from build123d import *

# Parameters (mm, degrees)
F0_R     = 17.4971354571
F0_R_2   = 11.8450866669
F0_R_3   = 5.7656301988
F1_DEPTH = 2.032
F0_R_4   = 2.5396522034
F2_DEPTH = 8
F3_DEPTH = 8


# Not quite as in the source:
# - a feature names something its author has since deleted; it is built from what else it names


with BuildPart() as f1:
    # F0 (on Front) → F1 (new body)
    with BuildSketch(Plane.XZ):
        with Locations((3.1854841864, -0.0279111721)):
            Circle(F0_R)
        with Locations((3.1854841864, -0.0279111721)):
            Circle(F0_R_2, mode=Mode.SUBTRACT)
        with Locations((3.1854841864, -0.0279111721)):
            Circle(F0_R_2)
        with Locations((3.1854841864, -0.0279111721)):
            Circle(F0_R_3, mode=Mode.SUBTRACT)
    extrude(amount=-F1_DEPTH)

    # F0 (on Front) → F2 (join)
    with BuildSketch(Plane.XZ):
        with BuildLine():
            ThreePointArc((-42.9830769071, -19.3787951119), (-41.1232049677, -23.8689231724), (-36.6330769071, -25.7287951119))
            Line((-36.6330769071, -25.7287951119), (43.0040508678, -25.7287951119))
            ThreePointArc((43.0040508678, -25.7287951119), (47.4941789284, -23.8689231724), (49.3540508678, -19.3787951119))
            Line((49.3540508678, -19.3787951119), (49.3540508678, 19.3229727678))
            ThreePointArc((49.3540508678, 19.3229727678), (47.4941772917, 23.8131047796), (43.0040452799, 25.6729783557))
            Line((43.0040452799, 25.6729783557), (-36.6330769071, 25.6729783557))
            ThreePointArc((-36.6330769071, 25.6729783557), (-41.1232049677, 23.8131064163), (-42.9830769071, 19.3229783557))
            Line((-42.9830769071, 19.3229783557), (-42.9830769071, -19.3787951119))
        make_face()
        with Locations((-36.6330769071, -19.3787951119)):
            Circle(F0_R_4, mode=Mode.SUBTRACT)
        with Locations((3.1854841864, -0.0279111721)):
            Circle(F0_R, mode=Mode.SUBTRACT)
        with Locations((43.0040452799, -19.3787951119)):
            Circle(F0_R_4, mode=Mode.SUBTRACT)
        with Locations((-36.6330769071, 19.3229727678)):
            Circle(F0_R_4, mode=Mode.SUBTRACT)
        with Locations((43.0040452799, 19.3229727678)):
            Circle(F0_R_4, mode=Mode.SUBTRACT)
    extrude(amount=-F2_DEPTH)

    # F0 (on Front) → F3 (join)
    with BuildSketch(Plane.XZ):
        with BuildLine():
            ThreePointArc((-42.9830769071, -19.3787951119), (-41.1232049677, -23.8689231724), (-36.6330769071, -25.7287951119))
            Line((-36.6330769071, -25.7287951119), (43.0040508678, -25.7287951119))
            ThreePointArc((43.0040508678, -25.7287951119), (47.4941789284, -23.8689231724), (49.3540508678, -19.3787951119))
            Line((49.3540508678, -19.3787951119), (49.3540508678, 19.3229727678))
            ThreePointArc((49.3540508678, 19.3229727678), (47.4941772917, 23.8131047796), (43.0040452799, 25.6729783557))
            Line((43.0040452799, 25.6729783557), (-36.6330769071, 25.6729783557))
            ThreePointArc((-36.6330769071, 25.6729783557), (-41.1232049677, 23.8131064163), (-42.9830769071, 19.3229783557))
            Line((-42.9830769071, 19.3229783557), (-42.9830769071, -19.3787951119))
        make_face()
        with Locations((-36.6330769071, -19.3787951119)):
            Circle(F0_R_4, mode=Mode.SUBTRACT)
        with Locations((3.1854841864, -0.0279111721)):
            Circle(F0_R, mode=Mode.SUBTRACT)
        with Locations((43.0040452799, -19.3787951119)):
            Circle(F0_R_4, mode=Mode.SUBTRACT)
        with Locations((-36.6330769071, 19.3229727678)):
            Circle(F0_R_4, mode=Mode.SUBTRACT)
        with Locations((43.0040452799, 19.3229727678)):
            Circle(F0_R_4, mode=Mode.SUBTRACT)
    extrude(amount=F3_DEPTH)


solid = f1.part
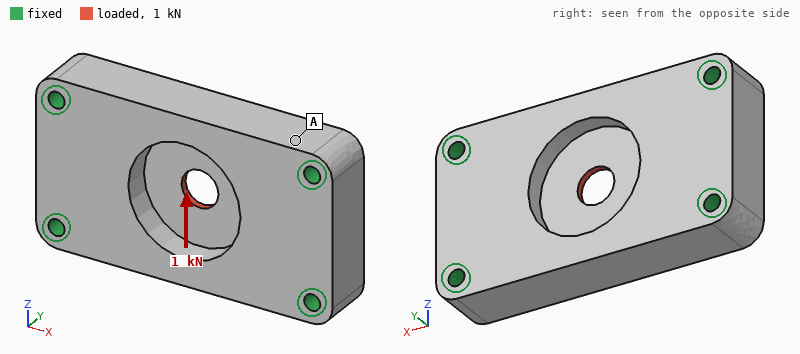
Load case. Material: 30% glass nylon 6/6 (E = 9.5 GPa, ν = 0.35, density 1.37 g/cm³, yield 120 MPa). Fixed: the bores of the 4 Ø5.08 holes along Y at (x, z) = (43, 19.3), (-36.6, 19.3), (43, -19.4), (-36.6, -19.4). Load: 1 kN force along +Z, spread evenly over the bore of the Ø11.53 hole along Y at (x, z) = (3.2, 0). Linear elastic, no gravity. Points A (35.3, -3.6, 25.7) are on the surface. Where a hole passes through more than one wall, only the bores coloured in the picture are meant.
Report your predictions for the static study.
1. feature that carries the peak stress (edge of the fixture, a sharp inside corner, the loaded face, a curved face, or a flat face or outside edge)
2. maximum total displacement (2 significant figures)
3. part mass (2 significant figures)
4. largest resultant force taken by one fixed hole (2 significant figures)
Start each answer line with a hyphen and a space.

- the loaded face
- 25 µm
- 83 g
- 350 N
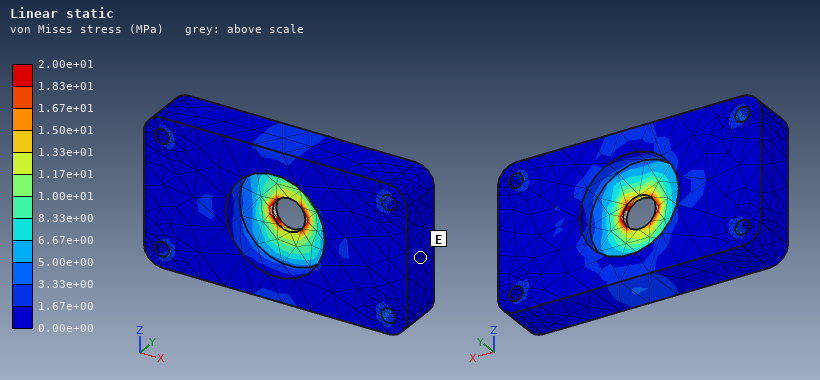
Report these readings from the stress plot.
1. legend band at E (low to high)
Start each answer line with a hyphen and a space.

- 0.00e+00 to 1.67e+00 MPa
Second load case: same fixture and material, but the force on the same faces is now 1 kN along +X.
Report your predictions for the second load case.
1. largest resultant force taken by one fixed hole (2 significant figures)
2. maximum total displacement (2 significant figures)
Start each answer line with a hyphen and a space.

- 260 N
- 18 µm
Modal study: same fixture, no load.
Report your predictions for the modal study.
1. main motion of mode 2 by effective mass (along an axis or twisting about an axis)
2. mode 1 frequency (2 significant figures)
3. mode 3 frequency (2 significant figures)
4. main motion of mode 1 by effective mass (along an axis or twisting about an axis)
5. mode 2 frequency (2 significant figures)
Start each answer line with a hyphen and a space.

- twisting about X
- 5300 Hz
- 9500 Hz
- along Y
- 6900 Hz
